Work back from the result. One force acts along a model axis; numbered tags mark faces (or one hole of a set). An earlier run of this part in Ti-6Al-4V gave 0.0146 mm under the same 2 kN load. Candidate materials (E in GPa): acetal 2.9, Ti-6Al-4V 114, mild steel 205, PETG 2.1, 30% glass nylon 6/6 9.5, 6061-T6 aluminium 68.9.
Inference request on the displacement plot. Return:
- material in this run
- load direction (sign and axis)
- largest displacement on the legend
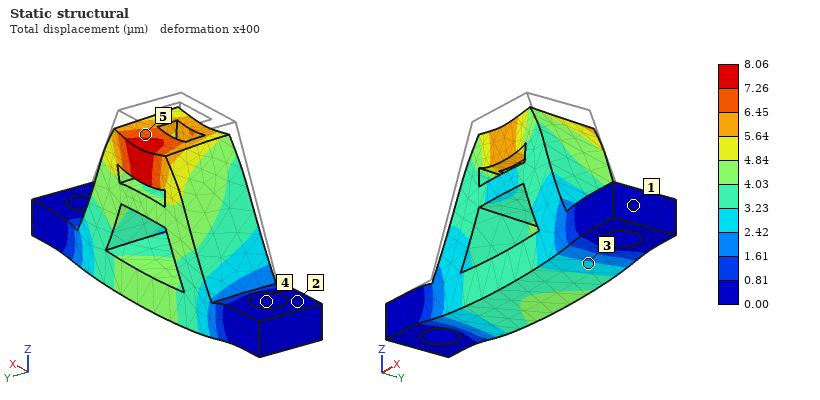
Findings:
mild steel
-Z
8.06 µm
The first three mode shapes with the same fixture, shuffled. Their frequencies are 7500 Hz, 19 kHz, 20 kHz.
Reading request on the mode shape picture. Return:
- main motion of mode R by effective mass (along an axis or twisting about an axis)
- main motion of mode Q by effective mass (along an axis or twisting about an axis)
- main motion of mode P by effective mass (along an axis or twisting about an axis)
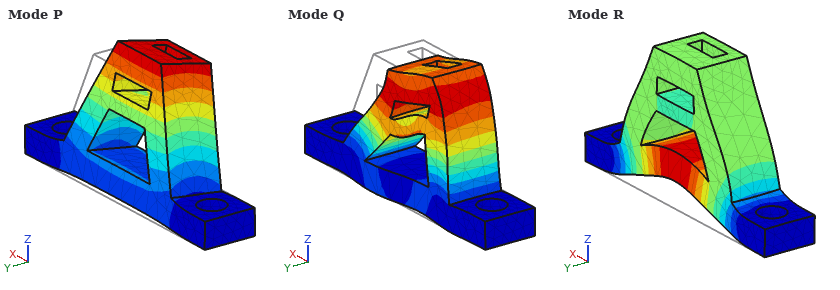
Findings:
along Z
along X
along Y
